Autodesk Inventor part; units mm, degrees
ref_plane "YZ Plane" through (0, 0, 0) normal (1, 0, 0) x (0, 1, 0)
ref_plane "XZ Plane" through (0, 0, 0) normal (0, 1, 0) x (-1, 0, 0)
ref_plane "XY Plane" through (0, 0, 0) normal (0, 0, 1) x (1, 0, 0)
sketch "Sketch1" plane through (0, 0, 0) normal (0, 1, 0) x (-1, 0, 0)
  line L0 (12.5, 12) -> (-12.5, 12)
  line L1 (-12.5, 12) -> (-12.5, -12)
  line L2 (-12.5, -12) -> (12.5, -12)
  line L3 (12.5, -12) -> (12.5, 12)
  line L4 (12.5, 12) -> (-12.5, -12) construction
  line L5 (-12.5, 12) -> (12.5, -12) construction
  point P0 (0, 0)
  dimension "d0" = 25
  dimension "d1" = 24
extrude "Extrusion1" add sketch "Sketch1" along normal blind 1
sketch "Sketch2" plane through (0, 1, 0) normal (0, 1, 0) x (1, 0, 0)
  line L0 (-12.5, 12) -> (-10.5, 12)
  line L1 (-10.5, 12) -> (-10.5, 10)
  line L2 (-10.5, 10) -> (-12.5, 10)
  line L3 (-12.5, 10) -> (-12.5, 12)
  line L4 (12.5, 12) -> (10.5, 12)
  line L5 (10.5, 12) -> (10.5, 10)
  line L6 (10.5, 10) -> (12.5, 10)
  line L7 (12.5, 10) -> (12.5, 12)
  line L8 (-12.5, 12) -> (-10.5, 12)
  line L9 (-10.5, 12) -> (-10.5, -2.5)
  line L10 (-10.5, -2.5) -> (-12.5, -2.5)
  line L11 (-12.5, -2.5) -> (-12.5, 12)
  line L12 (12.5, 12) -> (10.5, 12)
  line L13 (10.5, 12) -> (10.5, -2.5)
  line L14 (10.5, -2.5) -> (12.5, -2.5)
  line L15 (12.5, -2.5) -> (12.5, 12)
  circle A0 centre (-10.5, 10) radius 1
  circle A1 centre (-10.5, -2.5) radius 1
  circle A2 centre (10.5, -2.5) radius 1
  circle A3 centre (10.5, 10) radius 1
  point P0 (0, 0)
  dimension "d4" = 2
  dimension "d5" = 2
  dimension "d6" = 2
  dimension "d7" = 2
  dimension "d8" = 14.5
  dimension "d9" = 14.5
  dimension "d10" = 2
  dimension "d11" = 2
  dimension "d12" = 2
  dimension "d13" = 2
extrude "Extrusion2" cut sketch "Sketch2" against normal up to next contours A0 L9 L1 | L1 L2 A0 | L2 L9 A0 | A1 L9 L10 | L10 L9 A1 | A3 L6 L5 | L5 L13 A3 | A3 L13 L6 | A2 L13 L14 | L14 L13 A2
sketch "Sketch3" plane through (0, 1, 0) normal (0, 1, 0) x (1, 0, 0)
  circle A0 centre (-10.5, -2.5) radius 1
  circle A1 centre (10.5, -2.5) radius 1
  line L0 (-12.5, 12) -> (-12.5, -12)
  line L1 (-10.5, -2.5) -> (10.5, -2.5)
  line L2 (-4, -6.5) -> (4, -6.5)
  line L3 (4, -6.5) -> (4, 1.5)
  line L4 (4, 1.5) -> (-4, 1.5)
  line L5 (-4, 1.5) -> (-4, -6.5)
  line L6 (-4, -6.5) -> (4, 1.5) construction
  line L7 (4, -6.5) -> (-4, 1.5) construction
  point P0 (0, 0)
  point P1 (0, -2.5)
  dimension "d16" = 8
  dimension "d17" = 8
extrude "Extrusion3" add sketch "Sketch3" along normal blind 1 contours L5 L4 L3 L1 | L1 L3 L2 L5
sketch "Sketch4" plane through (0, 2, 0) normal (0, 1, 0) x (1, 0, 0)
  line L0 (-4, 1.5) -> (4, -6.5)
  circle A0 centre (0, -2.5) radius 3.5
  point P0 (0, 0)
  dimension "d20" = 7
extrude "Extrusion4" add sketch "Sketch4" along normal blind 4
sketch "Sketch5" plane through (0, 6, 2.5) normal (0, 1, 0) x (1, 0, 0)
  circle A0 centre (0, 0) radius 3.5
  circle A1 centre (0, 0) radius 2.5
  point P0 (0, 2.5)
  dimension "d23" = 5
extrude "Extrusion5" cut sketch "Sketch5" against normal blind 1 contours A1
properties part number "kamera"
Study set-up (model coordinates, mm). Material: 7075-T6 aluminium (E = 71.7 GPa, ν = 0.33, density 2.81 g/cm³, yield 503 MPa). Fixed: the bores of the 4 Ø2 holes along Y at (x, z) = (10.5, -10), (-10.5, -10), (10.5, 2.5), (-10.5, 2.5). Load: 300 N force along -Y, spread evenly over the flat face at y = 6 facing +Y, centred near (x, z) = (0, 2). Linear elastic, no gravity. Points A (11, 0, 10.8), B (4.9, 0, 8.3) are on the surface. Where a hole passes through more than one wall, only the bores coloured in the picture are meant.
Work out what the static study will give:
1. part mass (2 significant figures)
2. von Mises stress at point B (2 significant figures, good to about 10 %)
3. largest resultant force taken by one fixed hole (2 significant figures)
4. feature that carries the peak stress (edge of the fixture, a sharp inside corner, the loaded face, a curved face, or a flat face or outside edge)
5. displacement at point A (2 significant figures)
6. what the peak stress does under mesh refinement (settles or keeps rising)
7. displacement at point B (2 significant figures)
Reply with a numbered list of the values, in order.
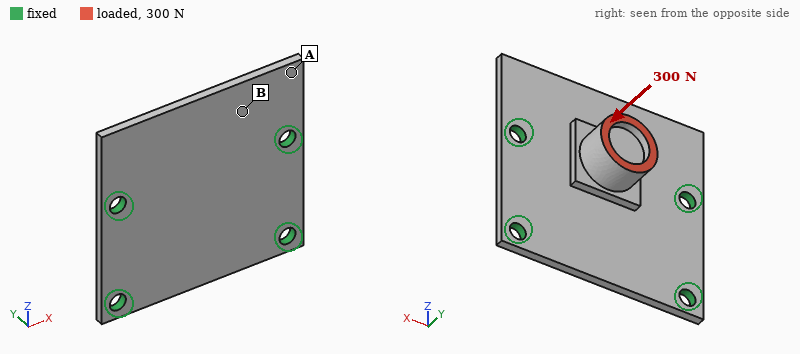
1. 2.2 g
2. 73 MPa
3. 160 N
4. edge of the fixture
5. 0.030 mm
6. keeps rising
7. 0.075 mm
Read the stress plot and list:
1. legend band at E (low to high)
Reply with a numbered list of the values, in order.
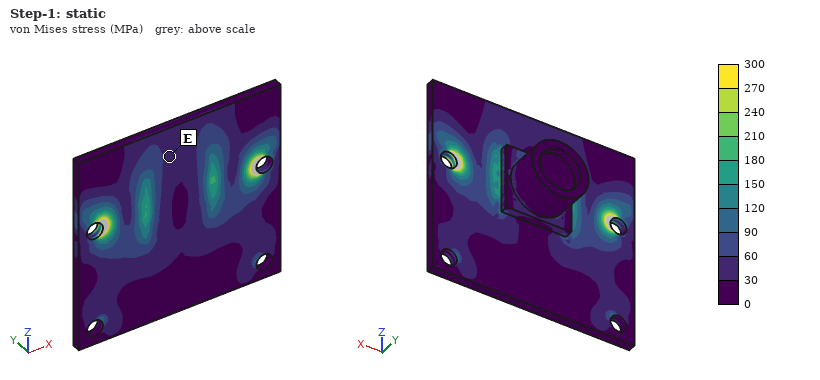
1. 30 to 60 MPa
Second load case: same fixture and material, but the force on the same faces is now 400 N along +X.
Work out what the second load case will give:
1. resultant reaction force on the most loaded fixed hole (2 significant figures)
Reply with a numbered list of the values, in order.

1. 200 N
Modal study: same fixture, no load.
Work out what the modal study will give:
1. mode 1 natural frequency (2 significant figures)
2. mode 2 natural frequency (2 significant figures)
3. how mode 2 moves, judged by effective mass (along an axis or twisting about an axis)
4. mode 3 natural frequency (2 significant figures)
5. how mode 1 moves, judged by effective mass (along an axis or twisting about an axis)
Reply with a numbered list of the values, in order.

1. 7700 Hz
2. 11 kHz
3. along Y
4. 14 kHz
5. along Y
